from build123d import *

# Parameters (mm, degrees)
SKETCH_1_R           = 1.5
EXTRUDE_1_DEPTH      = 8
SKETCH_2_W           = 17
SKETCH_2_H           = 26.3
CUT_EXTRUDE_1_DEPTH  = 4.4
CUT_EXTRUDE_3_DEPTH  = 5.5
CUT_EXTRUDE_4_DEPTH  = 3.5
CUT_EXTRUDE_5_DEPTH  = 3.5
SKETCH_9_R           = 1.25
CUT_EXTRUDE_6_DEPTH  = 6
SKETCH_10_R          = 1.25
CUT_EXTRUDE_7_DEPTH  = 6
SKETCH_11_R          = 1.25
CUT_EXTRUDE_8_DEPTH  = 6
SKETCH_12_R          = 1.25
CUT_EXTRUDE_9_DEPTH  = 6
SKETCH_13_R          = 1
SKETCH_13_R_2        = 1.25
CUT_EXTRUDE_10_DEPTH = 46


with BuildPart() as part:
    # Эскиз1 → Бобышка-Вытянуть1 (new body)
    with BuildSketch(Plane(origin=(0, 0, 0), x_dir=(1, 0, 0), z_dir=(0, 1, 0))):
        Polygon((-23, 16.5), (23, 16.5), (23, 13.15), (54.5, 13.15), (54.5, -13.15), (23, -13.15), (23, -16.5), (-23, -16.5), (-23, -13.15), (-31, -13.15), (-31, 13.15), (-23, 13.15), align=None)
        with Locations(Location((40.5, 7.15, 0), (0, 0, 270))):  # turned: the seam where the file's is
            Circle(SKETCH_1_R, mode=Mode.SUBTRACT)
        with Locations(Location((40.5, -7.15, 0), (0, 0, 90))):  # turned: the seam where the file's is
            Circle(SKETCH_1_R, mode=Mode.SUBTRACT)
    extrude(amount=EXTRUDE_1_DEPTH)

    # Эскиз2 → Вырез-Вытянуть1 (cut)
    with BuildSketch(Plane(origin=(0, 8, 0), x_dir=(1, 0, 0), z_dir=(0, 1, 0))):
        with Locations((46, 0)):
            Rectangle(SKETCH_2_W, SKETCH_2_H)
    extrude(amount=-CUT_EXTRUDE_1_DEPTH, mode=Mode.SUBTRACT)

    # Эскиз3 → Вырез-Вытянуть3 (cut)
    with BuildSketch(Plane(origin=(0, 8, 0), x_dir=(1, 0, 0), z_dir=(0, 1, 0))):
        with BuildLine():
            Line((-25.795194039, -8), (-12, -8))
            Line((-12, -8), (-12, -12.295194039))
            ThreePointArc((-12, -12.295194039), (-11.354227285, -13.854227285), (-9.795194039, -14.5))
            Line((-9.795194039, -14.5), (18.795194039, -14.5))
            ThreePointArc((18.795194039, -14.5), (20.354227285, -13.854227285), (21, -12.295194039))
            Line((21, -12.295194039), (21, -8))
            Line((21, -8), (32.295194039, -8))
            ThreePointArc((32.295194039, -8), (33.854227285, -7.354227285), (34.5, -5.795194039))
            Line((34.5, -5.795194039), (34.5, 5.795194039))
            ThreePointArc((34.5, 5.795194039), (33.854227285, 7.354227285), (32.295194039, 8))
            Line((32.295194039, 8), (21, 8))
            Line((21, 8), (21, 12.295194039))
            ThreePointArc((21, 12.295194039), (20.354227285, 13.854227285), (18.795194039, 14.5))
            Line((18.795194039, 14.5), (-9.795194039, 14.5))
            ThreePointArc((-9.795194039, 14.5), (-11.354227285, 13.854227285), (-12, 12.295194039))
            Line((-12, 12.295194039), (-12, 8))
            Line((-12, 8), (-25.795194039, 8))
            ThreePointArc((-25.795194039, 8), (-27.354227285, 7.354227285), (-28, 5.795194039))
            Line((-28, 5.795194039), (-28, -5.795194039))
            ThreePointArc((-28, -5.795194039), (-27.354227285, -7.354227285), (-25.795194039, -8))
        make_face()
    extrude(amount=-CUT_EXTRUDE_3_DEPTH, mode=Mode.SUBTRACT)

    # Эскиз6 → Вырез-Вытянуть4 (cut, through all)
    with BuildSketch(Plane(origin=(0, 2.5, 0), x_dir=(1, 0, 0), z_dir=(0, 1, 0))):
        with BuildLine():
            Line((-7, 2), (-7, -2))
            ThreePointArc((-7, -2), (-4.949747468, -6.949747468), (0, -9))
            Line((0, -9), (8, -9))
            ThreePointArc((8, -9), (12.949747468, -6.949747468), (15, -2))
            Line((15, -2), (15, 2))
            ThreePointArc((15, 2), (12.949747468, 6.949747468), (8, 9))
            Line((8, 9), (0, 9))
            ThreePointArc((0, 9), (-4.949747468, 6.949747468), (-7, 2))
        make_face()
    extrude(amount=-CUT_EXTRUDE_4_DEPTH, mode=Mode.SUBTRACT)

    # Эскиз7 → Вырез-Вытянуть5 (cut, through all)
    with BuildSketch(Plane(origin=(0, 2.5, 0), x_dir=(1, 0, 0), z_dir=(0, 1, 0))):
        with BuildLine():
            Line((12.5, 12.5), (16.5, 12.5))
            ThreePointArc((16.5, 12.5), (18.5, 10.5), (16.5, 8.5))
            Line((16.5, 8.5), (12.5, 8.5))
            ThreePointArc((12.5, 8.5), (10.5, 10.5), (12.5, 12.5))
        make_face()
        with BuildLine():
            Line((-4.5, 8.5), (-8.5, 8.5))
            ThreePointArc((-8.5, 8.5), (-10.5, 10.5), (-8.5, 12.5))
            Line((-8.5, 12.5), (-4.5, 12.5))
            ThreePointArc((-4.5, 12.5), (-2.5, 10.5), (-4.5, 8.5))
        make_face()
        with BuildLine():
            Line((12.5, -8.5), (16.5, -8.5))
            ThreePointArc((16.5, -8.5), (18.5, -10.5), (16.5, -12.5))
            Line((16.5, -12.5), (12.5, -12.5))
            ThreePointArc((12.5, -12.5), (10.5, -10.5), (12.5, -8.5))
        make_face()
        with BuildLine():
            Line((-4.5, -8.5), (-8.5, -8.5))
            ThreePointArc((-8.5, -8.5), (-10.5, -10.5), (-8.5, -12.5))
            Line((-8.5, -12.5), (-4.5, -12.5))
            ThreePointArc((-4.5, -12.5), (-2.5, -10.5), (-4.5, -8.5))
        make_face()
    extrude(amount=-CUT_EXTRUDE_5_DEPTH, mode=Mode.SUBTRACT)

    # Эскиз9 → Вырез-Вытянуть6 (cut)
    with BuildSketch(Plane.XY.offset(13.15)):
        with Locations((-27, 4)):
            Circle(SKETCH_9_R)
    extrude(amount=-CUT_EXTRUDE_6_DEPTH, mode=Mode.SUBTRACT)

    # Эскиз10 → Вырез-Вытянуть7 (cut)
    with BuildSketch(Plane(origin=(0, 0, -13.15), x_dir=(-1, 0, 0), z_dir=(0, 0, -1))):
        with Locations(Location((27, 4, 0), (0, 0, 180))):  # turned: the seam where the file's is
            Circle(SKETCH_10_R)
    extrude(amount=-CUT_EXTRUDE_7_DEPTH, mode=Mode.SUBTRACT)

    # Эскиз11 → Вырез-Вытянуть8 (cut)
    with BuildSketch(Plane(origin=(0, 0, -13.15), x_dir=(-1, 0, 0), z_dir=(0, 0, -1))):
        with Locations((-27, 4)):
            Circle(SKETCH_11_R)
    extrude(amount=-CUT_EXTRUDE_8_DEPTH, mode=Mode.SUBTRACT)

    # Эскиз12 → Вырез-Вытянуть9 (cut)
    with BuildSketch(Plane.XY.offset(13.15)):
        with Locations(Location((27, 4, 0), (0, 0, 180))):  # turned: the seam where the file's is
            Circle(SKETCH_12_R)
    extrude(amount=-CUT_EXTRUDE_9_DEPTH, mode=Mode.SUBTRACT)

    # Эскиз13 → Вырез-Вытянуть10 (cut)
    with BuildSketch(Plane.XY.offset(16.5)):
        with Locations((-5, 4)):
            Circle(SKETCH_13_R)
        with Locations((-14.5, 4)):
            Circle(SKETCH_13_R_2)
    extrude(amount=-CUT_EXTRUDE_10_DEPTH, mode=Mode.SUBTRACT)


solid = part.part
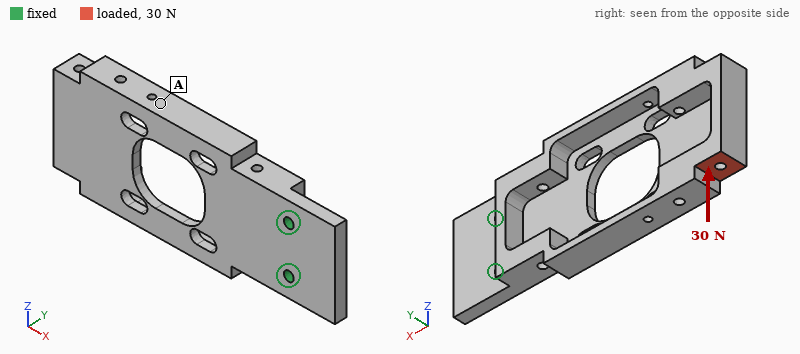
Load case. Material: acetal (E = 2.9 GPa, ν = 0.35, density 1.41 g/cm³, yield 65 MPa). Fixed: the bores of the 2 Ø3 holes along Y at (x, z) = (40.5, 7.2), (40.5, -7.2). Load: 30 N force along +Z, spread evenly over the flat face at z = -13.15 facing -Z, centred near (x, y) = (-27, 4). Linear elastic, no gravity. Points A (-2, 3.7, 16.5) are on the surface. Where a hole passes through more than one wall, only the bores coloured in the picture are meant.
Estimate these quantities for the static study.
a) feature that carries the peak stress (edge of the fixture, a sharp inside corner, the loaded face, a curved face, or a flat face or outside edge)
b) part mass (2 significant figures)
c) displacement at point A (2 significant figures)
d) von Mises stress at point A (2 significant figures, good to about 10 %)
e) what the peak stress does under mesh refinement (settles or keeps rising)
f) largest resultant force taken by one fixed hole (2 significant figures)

a sharp inside corner
13 g
0.34 mm
1.9 MPa
keeps rising
130 N
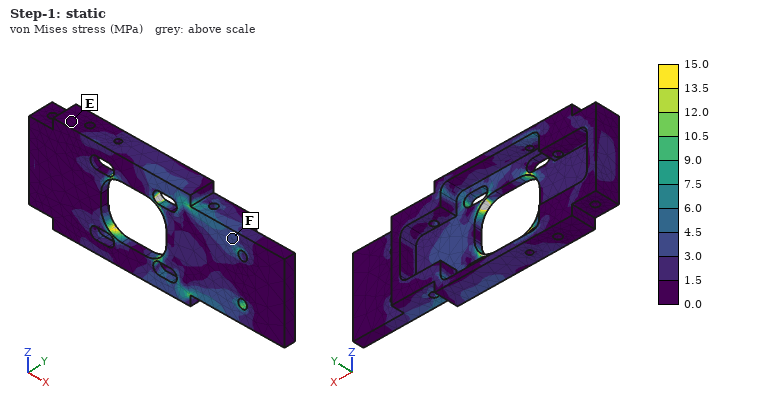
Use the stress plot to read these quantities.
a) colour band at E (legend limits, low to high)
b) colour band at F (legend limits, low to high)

0.0 to 1.5 MPa
3.0 to 4.5 MPa
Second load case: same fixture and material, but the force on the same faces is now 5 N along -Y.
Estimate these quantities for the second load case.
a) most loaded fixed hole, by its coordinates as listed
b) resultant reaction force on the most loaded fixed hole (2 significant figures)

(40.5, -7.2)
7.6 N
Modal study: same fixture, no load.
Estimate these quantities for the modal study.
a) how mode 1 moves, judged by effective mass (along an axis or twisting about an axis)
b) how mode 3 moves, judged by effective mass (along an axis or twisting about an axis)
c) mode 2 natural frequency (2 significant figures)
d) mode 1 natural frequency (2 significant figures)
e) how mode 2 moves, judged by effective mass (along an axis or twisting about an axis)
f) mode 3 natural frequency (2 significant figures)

along Y
along Z
510 Hz
190 Hz
along Z
750 Hz
